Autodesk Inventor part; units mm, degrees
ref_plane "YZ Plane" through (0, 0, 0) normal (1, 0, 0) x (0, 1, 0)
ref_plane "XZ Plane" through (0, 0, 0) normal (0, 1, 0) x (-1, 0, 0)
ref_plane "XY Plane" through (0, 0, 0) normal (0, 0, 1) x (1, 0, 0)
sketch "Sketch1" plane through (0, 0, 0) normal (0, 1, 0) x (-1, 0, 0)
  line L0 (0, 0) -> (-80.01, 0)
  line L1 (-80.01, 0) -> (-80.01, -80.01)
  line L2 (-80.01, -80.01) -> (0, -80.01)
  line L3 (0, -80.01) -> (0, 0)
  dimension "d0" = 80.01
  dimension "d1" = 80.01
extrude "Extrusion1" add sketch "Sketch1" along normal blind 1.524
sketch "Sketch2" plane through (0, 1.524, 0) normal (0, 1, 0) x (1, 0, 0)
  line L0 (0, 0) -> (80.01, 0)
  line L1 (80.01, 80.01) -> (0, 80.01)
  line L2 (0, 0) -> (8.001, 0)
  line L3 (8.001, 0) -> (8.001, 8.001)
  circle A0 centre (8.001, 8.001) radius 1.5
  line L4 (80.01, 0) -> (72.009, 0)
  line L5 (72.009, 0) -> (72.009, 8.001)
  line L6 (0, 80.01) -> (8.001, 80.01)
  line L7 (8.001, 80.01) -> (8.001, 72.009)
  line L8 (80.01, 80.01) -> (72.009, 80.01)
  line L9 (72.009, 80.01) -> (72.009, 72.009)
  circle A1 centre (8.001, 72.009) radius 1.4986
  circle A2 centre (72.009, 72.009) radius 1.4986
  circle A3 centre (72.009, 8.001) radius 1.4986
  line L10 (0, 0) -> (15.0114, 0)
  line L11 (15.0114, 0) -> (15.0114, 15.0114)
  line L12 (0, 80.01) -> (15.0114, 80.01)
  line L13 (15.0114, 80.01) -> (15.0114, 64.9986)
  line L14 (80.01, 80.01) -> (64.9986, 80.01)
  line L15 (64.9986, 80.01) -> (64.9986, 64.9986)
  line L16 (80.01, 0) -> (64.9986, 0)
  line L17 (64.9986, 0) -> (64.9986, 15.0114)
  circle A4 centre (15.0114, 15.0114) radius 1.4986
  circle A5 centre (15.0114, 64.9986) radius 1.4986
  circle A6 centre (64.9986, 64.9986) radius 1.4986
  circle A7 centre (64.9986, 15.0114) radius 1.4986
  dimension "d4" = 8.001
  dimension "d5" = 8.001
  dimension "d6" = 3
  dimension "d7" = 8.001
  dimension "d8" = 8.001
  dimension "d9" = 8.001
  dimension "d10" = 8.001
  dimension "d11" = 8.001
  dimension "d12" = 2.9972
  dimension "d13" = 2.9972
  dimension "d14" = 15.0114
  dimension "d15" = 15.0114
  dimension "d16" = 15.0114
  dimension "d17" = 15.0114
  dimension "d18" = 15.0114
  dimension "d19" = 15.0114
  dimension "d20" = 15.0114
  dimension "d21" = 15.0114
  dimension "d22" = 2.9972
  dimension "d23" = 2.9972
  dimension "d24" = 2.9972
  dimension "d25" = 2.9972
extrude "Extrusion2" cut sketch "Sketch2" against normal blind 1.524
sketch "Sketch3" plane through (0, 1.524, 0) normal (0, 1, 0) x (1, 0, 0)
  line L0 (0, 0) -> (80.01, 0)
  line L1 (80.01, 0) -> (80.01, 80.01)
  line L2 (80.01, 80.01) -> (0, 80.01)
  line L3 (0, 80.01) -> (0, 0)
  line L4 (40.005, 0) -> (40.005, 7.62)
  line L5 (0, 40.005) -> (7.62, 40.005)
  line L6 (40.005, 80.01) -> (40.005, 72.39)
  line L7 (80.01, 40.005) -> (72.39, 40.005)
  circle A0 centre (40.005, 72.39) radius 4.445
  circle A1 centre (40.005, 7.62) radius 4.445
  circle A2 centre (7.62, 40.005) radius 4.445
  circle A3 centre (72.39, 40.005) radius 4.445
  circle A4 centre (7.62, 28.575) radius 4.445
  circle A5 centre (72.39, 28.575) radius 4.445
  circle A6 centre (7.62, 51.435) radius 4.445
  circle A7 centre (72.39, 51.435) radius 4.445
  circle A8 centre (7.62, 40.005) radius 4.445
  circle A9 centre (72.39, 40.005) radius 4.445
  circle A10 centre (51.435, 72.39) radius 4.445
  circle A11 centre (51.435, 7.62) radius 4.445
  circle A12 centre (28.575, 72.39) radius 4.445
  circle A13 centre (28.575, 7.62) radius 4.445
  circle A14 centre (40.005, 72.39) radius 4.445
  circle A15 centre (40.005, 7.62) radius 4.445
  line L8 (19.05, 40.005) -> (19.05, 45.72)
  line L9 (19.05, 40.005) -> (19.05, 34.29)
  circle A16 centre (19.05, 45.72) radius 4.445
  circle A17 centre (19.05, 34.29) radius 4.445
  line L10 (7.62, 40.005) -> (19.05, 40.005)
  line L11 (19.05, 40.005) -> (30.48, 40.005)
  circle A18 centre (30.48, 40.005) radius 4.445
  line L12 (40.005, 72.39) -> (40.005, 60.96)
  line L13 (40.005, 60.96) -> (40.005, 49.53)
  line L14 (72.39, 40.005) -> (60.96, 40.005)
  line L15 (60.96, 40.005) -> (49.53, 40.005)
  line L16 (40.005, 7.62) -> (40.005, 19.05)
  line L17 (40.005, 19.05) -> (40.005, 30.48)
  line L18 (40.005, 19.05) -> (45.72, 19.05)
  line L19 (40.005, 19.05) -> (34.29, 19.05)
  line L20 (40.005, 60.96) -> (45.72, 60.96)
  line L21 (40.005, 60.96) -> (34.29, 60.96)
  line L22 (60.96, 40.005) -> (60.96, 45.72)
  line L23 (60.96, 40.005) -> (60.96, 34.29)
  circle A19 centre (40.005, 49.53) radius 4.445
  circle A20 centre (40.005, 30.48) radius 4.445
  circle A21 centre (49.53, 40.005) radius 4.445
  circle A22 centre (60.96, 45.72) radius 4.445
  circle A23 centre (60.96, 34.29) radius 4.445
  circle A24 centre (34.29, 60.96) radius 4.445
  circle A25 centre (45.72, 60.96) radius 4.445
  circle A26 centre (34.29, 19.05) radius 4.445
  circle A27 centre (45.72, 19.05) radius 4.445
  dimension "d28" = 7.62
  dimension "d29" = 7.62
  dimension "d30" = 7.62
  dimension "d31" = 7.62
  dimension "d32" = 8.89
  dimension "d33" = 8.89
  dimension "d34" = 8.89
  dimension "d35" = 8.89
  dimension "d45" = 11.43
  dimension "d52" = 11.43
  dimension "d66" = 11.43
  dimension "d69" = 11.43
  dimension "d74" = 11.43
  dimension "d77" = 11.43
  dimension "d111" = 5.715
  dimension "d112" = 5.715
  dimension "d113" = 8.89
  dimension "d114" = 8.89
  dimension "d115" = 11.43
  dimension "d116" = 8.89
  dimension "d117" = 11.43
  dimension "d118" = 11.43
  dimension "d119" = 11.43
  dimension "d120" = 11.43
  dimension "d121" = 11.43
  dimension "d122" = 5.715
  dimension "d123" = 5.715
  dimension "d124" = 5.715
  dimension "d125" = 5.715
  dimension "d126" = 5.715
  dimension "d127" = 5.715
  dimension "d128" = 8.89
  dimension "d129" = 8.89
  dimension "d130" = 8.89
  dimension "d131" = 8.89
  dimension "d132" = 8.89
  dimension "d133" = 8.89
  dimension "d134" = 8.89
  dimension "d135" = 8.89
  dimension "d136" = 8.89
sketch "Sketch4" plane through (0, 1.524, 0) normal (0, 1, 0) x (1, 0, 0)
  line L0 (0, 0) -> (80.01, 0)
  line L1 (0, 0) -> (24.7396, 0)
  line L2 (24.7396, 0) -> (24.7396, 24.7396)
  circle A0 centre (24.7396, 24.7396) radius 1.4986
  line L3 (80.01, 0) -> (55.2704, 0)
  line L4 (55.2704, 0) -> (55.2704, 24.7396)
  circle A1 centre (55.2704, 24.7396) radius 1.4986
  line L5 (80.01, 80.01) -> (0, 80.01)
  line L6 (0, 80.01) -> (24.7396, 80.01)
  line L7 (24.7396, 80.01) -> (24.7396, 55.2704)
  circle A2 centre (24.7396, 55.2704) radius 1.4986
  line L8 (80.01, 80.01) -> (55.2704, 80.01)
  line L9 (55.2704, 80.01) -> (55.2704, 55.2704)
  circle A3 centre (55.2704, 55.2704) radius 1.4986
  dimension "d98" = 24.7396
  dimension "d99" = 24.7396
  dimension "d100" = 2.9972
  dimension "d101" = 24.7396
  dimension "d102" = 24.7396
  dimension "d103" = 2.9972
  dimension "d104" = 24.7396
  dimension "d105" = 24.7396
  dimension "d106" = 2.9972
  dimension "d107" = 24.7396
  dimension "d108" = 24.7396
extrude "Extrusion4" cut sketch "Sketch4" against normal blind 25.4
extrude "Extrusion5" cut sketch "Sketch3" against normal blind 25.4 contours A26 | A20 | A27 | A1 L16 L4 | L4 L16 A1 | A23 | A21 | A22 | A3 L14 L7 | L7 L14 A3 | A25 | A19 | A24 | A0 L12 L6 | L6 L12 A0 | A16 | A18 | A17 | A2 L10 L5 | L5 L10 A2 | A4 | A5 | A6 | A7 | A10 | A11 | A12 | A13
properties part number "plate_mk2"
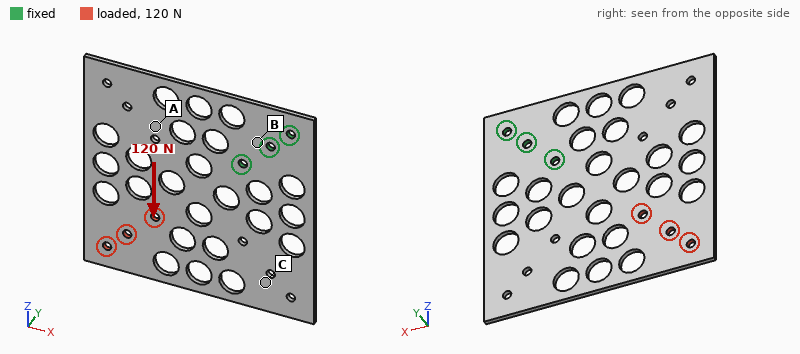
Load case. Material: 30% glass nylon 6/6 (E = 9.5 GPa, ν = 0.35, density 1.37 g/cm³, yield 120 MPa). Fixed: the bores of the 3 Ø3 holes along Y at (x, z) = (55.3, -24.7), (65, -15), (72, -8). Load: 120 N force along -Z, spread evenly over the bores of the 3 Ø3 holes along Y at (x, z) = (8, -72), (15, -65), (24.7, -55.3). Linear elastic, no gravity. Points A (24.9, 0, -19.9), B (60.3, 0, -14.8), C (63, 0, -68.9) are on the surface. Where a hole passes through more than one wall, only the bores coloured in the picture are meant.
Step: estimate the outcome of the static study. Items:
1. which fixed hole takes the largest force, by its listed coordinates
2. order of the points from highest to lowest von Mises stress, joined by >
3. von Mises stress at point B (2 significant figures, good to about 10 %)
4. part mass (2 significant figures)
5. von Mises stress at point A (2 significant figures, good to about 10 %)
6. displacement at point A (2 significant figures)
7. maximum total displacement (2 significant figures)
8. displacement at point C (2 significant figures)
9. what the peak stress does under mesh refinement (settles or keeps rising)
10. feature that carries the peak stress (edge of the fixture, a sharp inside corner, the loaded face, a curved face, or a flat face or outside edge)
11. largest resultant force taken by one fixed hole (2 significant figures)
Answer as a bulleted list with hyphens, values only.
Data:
- (55.3, -24.7)
- B > A > C
- 6.6 MPa
- 10 g
- 4.8 MPa
- 0.14 mm
- 0.33 mm
- 0.17 mm
- keeps rising
- edge of the fixture
- 280 N
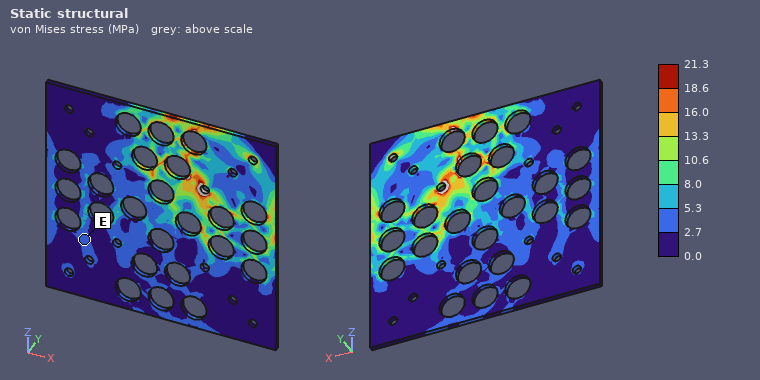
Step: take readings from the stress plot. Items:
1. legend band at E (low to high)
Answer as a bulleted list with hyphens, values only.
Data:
- 2.7 to 5.3 MPa
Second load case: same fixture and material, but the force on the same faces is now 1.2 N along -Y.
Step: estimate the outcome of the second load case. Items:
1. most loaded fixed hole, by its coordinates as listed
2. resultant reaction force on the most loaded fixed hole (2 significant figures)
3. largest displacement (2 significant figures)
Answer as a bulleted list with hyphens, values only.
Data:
- (55.3, -24.7)
- 3.3 N
- 1.2 mm
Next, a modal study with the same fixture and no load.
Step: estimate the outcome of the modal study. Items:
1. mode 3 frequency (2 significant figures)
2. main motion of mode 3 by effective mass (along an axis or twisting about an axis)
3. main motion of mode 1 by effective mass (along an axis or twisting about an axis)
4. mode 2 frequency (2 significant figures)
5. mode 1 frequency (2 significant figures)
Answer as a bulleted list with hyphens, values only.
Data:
- 310 Hz
- along Y
- along Y
- 170 Hz
- 120 Hz
